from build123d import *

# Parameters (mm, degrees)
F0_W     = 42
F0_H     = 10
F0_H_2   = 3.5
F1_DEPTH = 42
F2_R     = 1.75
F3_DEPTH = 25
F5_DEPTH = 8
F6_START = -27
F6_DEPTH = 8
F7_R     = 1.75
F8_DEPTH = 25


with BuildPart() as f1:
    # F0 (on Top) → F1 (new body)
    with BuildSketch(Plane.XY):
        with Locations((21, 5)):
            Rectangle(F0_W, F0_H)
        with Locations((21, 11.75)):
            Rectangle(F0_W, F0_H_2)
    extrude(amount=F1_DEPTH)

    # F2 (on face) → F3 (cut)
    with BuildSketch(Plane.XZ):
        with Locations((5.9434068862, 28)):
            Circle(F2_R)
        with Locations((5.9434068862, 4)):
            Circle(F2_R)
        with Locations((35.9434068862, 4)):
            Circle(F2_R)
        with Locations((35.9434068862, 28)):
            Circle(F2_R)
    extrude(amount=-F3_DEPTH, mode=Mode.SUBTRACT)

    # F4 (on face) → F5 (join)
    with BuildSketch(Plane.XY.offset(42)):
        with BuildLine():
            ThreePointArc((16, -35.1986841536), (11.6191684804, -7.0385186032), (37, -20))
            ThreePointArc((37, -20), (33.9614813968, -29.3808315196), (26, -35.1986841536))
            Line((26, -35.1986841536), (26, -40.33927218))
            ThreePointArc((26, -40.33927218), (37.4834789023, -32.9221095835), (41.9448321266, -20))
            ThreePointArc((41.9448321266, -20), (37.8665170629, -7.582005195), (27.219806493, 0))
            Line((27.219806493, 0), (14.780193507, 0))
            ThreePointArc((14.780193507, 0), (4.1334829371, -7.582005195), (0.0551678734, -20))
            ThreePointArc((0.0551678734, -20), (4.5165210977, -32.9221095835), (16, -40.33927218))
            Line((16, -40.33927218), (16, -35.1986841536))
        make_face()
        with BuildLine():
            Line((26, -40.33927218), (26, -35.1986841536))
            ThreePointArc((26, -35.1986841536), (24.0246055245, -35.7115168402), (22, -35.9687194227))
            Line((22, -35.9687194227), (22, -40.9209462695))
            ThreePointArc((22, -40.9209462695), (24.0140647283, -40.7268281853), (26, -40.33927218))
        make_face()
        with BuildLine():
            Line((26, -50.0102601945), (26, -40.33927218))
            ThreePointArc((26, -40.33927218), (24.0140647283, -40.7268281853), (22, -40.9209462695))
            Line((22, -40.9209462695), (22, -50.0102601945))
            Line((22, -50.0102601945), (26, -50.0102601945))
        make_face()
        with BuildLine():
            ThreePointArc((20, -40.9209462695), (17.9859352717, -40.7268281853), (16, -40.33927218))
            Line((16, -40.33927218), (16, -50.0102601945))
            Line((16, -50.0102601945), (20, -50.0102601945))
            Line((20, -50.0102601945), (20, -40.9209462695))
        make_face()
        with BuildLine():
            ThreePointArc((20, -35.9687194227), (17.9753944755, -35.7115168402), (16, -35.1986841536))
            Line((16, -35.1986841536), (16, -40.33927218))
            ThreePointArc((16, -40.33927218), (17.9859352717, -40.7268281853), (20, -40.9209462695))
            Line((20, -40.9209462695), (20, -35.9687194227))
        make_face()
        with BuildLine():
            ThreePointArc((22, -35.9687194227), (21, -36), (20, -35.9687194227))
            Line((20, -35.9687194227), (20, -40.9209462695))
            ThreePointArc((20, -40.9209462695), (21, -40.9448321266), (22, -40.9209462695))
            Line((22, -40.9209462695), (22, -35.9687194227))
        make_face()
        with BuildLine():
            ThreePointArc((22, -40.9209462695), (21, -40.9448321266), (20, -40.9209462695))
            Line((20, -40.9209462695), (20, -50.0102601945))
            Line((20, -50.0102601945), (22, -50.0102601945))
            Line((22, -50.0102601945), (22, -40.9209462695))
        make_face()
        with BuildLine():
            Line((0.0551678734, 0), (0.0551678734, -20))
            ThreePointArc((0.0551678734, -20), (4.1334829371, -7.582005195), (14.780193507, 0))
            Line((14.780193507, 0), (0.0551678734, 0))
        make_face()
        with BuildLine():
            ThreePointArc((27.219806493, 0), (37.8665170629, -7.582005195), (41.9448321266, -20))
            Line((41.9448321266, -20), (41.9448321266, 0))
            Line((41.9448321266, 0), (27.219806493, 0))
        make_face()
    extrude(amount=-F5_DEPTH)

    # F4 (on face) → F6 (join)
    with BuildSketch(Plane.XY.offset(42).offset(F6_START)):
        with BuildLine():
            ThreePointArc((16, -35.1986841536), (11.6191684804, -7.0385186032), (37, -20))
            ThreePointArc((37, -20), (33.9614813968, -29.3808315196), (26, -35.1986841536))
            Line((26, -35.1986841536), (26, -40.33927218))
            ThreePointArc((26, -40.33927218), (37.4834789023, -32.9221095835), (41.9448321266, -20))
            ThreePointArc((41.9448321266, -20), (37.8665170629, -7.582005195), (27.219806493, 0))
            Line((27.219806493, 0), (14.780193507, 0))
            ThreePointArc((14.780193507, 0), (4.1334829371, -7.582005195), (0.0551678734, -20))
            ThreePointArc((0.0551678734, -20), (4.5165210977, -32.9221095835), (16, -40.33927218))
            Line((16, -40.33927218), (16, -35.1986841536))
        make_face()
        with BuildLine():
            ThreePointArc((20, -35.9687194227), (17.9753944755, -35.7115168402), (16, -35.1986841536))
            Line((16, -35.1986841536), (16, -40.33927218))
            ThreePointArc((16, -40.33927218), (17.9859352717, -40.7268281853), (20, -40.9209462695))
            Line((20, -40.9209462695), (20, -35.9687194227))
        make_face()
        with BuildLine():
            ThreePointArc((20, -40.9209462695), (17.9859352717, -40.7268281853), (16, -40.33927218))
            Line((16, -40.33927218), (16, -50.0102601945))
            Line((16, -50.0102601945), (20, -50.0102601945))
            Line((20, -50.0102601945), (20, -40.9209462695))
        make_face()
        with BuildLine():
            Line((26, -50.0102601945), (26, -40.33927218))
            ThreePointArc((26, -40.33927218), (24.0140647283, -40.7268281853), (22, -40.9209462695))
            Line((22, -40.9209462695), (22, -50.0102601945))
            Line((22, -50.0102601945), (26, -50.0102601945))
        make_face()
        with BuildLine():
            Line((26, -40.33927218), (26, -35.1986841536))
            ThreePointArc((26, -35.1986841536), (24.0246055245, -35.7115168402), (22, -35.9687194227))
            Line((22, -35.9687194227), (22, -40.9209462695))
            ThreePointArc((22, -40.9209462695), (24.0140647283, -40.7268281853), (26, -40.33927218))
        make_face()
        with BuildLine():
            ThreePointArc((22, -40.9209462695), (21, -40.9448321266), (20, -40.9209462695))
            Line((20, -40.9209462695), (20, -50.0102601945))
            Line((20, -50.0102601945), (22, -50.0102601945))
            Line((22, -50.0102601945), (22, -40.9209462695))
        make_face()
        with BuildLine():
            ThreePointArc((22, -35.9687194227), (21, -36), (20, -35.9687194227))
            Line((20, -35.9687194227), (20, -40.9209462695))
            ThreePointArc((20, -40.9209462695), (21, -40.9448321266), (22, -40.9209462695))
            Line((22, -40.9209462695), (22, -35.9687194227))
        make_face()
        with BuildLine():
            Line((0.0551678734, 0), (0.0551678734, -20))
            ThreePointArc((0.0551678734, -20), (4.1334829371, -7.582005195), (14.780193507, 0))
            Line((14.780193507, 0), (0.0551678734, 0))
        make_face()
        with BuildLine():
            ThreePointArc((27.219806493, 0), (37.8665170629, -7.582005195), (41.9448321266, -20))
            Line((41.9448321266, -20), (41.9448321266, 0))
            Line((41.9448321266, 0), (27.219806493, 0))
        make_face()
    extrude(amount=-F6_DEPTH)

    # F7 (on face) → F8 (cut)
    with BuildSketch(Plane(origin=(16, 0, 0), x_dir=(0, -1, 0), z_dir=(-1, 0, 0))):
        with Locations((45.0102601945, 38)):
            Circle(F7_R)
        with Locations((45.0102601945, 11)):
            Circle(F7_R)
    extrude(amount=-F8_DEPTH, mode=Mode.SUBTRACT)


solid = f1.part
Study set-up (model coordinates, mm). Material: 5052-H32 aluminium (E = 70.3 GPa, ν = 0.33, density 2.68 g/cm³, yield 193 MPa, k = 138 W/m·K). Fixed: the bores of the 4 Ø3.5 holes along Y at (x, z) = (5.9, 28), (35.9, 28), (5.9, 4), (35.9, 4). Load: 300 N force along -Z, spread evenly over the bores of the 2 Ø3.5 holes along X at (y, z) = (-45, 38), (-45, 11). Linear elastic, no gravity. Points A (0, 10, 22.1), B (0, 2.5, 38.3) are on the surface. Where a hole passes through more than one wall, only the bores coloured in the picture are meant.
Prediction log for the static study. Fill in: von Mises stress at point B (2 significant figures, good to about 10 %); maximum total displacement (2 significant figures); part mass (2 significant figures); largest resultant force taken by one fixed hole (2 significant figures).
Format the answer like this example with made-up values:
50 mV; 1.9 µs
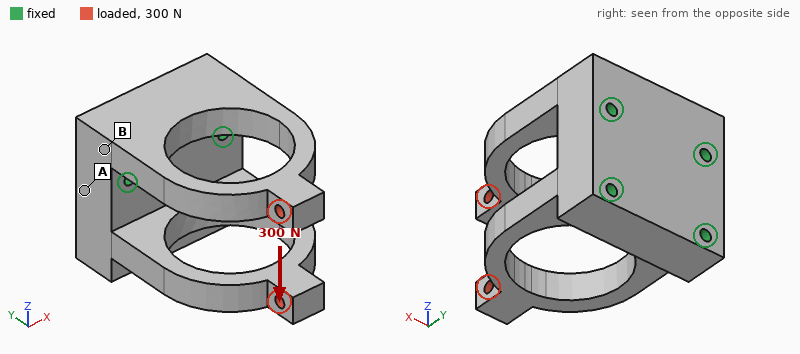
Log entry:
10 MPa; 0.18 mm; 97 g; 230 N
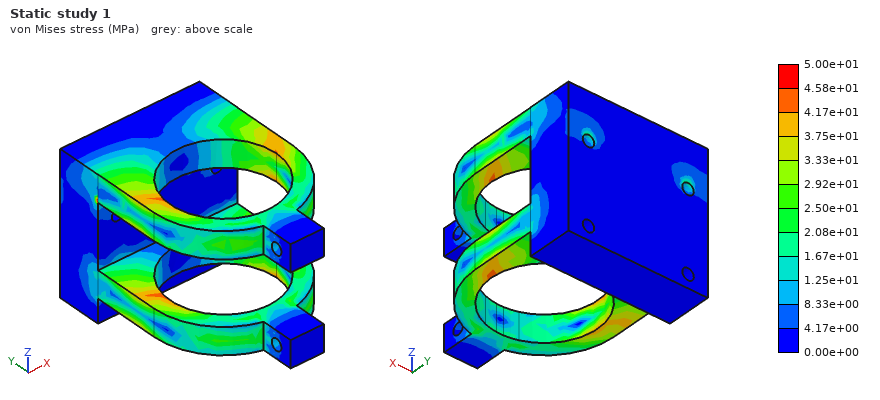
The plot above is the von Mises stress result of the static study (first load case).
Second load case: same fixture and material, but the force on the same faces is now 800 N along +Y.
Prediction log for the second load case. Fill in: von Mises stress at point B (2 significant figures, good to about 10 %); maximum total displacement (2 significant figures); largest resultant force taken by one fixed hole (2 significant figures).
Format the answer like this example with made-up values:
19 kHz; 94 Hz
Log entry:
6.3 MPa; 17 µm; 270 N
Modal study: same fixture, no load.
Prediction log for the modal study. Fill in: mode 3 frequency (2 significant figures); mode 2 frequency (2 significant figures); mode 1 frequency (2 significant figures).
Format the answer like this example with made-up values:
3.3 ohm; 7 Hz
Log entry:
5200 Hz; 2700 Hz; 2600 Hz
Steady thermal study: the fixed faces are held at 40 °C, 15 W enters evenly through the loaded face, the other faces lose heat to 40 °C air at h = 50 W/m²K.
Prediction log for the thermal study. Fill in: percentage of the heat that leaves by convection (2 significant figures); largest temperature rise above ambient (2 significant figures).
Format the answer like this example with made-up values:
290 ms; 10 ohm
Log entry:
26 %; 28 K
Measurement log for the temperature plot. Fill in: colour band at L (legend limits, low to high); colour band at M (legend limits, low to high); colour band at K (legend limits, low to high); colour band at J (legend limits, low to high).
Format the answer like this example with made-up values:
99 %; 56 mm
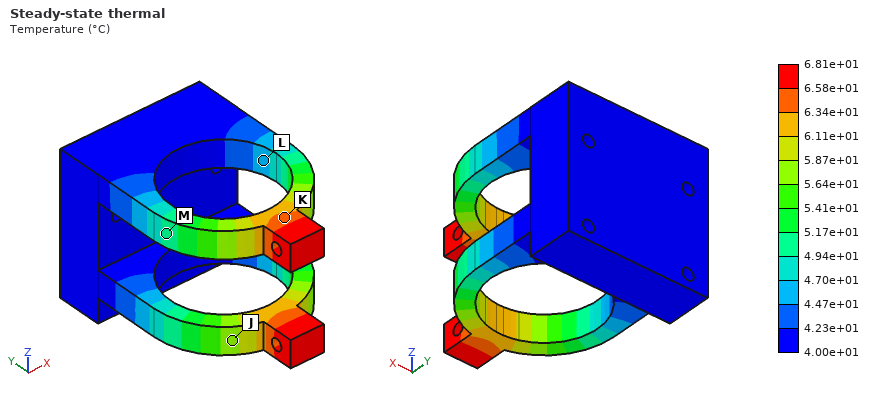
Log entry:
4.47e+01 to 4.70e+01 °C; 4.94e+01 to 5.17e+01 °C; 6.34e+01 to 6.58e+01 °C; 5.64e+01 to 5.87e+01 °C
